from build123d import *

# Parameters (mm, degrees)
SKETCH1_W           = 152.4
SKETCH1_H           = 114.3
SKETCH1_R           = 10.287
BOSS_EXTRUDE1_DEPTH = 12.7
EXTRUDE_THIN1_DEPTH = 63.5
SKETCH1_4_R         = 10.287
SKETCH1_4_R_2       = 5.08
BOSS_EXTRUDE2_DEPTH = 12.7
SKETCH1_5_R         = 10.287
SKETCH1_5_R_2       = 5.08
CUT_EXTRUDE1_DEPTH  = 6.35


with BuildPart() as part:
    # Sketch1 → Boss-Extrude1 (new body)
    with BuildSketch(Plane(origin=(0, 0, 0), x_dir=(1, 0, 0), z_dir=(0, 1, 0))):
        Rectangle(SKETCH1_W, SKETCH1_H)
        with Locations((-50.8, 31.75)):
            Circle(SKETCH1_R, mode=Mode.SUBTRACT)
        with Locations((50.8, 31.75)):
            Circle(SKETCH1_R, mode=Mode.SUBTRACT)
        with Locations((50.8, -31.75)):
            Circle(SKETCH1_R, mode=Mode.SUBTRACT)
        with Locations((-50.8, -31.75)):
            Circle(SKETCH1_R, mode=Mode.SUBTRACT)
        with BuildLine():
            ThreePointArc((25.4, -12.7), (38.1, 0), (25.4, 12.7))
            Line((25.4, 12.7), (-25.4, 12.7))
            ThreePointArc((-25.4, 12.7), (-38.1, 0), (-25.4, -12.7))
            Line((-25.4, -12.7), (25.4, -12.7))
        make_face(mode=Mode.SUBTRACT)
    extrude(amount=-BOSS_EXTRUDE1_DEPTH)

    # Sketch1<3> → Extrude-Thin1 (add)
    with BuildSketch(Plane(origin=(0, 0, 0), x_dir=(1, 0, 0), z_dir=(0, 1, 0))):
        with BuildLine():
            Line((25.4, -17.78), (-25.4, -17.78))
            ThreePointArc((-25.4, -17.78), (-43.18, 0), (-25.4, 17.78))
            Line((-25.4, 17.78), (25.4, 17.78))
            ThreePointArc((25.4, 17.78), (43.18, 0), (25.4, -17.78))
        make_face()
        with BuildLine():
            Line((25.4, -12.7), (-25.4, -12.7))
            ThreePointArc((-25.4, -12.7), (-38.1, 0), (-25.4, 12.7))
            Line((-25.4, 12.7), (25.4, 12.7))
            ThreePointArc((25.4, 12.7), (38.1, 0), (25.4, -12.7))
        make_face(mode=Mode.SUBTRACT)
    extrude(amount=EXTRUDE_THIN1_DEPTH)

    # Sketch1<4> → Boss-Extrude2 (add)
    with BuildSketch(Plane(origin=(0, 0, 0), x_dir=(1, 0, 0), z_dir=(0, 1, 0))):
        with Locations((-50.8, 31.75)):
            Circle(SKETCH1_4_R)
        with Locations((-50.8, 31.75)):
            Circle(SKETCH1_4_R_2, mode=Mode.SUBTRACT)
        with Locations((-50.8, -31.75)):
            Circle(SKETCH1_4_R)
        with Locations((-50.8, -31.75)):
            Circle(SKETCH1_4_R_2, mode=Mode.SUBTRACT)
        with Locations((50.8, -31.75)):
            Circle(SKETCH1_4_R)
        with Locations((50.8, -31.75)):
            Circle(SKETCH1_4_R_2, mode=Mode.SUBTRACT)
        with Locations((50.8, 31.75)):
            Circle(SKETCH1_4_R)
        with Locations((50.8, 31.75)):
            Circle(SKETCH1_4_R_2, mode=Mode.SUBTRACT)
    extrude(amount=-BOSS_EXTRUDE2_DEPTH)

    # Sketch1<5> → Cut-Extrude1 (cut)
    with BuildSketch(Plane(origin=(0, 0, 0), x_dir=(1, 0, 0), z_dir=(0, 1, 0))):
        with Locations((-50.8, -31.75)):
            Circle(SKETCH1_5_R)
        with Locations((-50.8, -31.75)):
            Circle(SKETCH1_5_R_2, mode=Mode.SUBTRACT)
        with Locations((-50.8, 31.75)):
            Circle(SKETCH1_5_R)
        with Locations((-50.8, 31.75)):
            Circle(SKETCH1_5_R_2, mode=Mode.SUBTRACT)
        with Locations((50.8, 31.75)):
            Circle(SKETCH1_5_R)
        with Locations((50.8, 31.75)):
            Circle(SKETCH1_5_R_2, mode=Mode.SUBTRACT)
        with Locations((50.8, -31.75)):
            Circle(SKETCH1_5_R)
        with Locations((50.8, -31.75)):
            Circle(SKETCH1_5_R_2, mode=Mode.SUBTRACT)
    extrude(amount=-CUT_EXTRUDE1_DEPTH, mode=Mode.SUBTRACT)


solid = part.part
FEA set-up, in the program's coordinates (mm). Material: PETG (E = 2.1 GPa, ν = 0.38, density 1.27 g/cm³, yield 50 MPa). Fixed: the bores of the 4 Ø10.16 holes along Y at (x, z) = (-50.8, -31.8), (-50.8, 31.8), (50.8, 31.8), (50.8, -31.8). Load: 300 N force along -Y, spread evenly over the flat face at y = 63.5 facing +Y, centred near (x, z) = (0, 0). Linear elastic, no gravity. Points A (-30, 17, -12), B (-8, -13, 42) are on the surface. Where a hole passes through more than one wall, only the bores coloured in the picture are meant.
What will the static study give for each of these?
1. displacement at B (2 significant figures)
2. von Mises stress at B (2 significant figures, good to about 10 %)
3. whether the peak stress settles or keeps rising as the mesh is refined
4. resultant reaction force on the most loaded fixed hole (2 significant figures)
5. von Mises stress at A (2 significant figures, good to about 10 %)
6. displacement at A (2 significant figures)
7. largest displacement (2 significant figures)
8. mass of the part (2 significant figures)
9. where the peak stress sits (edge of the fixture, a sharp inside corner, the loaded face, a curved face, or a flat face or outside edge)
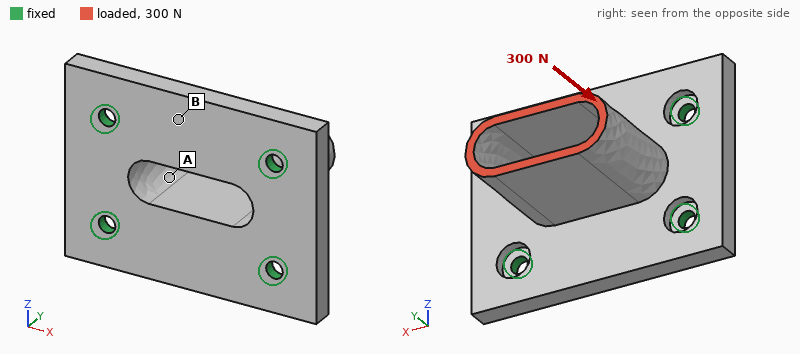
14 µm
0.16 MPa
keeps rising
110 N
0.53 MPa
31 µm
40 µm
320 g
edge of the fixture
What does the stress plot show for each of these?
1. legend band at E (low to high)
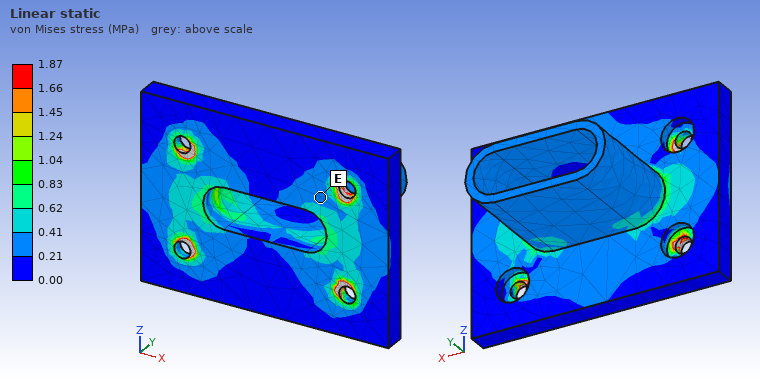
0.21 to 0.41 MPa
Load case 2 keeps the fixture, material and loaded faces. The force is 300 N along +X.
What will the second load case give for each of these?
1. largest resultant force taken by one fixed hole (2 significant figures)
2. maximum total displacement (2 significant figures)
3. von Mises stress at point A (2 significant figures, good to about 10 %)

160 N
0.15 mm
1.0 MPa
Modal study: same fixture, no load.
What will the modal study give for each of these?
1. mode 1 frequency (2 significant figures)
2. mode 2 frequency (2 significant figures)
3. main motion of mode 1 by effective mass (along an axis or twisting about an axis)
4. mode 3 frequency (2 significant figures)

680 Hz
960 Hz
along Z
1100 Hz
